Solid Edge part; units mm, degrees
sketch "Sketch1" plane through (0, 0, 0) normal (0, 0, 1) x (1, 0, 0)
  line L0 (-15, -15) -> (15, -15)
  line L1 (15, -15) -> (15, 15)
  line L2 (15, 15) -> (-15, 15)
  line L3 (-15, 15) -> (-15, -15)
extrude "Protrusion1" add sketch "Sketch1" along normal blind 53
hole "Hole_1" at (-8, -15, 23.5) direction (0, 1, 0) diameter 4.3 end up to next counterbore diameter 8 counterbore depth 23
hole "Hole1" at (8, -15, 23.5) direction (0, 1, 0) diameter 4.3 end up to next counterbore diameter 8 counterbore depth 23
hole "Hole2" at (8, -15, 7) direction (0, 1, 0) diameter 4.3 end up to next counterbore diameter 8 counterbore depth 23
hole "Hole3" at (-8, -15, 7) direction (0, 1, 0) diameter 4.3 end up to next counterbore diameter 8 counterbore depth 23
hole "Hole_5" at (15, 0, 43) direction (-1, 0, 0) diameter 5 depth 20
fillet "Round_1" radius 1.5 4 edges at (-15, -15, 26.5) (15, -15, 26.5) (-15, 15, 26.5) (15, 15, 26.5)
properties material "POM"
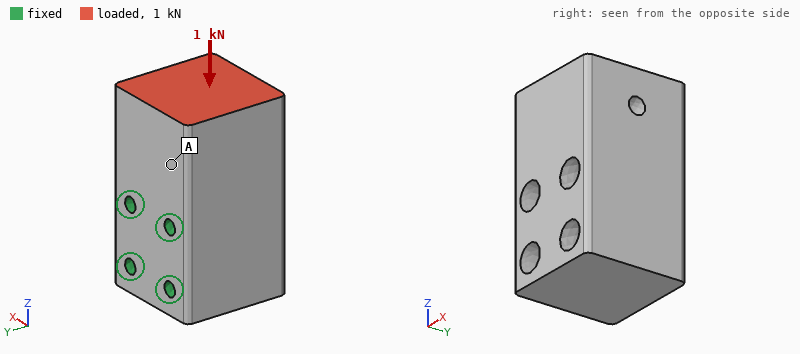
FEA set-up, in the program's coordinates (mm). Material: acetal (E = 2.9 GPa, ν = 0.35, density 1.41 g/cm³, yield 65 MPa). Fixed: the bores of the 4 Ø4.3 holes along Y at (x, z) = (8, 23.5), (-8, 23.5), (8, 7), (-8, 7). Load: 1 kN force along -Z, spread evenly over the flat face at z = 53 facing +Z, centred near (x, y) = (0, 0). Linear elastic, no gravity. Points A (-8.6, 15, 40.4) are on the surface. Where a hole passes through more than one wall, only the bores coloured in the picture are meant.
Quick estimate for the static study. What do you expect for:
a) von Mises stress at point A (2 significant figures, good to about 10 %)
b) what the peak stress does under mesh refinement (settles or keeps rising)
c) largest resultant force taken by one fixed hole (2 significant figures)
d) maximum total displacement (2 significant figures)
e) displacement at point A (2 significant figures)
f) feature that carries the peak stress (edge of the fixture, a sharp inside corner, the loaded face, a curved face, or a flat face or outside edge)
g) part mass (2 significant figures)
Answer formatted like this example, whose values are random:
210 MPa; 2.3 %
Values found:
1.3 MPa; keeps rising; 410 N; 0.10 mm; 0.041 mm; edge of the fixture; 59 g
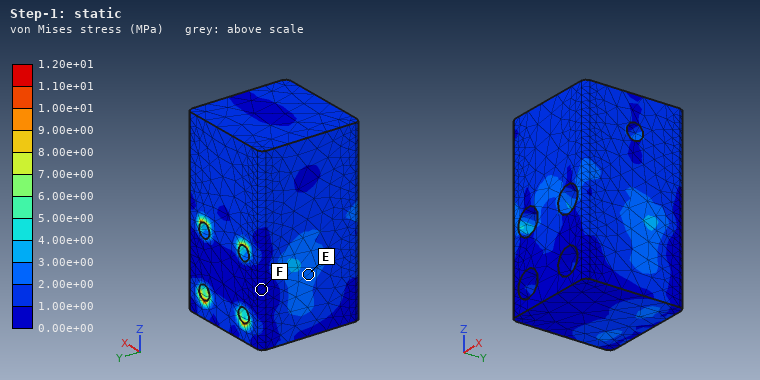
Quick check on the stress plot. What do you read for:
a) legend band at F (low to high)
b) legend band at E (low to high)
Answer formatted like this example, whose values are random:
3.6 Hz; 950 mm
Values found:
0.00e+00 to 1.00e+00 MPa; 2.00e+00 to 3.00e+00 MPa
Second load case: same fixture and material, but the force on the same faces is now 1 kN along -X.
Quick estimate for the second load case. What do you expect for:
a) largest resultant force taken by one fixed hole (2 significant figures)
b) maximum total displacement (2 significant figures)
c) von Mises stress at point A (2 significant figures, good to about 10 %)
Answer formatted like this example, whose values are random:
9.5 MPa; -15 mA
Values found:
1.2 kN; 0.24 mm; 3.5 MPa
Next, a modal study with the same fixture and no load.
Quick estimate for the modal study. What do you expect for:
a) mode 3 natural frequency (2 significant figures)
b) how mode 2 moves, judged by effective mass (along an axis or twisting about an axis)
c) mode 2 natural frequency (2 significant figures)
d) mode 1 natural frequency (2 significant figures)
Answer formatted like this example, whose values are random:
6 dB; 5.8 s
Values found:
3900 Hz; along X; 2700 Hz; 2100 Hz
